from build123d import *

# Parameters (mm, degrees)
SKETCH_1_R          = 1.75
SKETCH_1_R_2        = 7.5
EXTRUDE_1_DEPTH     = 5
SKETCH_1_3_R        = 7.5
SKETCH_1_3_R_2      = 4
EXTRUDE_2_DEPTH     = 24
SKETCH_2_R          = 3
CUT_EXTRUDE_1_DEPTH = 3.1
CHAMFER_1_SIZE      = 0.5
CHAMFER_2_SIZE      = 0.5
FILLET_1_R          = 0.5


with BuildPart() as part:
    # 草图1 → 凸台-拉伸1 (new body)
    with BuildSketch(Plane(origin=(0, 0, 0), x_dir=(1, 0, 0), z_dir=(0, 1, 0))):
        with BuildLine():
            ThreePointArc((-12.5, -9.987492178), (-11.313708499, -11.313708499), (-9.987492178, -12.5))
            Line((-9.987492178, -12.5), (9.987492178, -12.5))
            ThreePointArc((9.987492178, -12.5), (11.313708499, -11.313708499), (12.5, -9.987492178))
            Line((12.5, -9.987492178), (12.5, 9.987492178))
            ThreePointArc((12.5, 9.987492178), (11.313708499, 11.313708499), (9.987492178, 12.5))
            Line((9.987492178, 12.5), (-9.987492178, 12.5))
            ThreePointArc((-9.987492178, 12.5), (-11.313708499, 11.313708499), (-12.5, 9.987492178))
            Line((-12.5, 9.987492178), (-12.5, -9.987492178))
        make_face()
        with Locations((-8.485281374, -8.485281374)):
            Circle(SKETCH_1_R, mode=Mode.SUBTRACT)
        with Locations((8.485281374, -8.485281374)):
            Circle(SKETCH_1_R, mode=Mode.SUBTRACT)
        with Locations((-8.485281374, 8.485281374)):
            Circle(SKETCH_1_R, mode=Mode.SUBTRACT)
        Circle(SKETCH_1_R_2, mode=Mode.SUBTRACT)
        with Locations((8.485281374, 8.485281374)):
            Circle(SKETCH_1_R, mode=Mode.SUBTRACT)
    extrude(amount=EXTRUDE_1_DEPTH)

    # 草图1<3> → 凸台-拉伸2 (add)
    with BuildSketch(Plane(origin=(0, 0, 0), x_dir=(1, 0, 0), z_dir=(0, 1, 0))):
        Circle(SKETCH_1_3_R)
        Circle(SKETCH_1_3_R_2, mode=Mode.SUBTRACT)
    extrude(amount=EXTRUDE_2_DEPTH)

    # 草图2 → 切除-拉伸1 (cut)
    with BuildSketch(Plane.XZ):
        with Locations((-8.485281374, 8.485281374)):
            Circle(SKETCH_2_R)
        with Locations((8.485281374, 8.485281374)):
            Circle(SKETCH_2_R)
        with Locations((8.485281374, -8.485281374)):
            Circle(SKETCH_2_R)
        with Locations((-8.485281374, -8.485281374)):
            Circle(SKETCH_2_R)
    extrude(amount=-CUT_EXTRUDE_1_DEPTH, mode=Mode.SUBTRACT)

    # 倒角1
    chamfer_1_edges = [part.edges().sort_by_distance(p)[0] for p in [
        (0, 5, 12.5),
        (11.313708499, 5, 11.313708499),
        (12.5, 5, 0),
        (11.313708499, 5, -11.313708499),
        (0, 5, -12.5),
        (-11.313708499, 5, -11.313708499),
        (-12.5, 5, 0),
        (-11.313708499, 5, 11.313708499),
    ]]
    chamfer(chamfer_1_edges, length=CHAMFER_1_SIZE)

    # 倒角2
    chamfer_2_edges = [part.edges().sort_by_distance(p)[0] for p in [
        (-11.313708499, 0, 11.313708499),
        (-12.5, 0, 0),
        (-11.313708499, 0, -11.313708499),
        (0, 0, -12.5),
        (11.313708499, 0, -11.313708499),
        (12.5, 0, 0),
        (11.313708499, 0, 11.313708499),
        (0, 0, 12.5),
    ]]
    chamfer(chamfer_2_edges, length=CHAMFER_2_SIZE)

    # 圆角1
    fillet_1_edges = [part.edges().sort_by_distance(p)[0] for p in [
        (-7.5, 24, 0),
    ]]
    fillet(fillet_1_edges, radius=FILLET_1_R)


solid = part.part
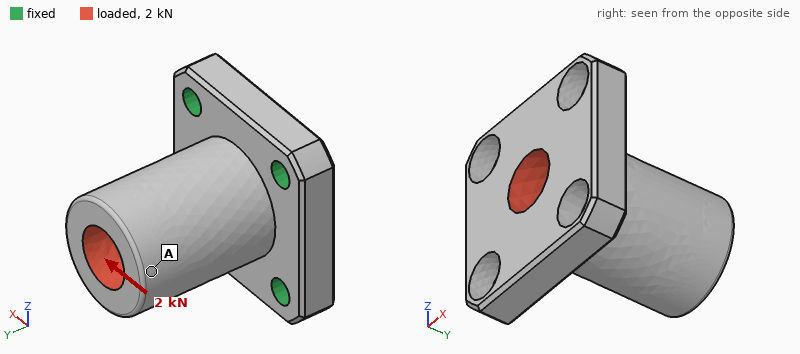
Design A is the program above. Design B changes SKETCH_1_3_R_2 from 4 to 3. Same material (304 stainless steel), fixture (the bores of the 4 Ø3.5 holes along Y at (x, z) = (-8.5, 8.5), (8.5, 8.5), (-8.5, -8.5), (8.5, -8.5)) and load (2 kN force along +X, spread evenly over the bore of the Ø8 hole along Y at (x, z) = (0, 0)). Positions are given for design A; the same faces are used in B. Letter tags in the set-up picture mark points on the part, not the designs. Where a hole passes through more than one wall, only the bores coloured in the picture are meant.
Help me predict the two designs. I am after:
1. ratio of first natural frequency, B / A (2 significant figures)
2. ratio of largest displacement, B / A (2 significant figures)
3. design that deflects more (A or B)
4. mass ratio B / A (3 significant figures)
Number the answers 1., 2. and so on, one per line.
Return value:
1. 0.97
2. 0.92
3. A
4. 1.11
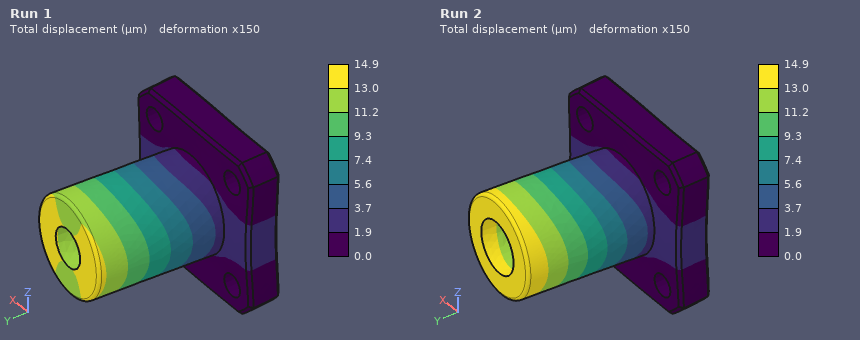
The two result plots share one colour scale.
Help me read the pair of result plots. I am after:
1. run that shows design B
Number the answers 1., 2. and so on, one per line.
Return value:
1. Run 1
